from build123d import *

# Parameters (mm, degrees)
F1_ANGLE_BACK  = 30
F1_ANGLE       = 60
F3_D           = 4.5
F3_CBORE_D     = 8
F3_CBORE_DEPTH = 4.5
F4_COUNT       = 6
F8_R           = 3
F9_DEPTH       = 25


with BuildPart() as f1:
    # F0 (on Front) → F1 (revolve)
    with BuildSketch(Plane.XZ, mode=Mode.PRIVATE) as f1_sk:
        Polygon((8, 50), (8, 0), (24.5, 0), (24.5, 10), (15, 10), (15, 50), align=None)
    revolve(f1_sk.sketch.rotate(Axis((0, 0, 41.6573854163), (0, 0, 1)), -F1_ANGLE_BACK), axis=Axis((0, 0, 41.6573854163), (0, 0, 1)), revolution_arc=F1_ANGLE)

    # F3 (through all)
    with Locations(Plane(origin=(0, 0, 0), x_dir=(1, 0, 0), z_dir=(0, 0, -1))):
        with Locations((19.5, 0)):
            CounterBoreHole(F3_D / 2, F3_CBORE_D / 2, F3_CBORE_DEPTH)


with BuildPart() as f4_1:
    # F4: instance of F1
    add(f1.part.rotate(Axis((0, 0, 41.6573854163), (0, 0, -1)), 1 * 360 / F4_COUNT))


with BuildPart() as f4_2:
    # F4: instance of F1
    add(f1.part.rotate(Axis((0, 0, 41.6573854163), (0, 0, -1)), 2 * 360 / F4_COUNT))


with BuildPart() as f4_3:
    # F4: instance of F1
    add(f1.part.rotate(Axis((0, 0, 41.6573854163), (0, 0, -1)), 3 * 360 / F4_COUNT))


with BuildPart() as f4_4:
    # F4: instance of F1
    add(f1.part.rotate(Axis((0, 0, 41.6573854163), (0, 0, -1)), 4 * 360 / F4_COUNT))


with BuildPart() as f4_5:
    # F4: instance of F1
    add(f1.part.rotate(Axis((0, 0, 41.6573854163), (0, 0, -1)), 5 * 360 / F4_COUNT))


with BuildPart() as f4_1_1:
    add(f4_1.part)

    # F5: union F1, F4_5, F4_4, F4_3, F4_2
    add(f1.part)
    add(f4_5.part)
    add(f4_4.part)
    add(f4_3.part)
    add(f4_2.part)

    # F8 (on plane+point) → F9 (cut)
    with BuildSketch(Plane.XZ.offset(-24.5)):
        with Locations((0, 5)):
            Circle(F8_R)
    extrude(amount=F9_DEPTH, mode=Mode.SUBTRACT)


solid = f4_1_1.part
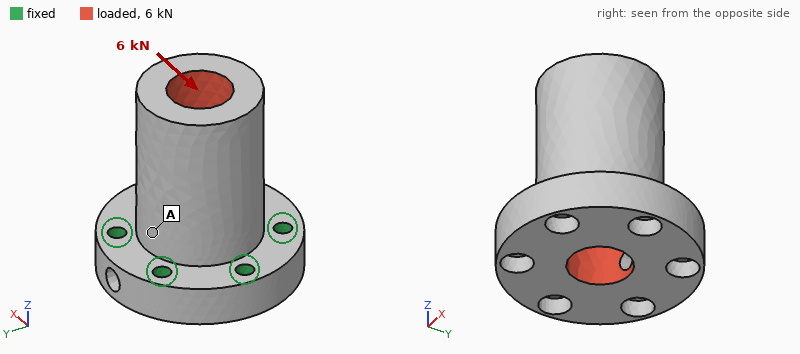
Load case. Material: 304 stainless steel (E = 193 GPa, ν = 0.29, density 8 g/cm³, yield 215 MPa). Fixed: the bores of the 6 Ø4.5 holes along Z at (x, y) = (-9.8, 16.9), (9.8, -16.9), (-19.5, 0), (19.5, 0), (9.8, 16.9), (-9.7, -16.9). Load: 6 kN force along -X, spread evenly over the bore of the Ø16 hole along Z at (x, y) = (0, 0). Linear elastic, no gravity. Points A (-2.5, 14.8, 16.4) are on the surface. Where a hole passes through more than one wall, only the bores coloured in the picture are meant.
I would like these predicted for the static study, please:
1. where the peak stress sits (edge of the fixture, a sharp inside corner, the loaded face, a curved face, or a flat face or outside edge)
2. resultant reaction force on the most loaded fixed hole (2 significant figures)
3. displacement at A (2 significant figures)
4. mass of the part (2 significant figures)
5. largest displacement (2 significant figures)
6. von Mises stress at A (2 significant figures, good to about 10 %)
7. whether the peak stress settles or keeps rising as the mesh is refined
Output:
edge of the fixture
2.4 kN
3.0 µm
280 g
17 µm
15 MPa
keeps rising
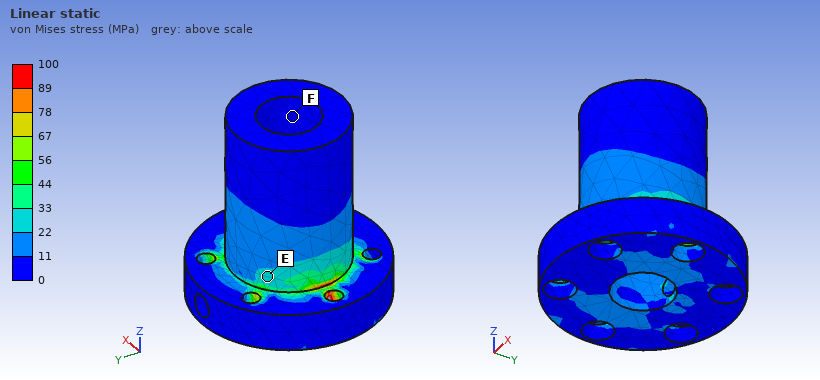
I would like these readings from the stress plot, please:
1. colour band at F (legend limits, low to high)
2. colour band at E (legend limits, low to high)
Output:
0 to 11 MPa
22 to 33 MPa
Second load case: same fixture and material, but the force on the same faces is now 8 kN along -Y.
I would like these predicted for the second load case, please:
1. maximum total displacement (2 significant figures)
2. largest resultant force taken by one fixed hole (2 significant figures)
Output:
23 µm
2.8 kN
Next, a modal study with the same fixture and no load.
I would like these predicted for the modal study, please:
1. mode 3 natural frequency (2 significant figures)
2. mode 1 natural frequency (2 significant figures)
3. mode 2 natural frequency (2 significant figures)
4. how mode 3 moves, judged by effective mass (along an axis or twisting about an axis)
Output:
17 kHz
7800 Hz
7900 Hz
twisting about Z
